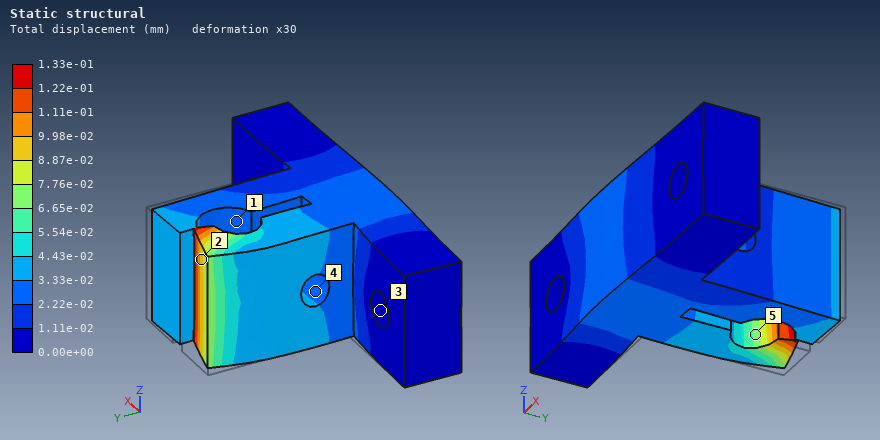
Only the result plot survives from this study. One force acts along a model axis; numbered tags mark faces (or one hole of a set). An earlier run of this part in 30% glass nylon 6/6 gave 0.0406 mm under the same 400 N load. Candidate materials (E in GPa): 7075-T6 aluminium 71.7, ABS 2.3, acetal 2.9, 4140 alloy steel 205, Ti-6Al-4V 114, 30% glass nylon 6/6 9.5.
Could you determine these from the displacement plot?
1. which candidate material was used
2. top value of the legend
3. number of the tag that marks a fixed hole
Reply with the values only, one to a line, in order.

acetal
1.33e-01 mm
3
